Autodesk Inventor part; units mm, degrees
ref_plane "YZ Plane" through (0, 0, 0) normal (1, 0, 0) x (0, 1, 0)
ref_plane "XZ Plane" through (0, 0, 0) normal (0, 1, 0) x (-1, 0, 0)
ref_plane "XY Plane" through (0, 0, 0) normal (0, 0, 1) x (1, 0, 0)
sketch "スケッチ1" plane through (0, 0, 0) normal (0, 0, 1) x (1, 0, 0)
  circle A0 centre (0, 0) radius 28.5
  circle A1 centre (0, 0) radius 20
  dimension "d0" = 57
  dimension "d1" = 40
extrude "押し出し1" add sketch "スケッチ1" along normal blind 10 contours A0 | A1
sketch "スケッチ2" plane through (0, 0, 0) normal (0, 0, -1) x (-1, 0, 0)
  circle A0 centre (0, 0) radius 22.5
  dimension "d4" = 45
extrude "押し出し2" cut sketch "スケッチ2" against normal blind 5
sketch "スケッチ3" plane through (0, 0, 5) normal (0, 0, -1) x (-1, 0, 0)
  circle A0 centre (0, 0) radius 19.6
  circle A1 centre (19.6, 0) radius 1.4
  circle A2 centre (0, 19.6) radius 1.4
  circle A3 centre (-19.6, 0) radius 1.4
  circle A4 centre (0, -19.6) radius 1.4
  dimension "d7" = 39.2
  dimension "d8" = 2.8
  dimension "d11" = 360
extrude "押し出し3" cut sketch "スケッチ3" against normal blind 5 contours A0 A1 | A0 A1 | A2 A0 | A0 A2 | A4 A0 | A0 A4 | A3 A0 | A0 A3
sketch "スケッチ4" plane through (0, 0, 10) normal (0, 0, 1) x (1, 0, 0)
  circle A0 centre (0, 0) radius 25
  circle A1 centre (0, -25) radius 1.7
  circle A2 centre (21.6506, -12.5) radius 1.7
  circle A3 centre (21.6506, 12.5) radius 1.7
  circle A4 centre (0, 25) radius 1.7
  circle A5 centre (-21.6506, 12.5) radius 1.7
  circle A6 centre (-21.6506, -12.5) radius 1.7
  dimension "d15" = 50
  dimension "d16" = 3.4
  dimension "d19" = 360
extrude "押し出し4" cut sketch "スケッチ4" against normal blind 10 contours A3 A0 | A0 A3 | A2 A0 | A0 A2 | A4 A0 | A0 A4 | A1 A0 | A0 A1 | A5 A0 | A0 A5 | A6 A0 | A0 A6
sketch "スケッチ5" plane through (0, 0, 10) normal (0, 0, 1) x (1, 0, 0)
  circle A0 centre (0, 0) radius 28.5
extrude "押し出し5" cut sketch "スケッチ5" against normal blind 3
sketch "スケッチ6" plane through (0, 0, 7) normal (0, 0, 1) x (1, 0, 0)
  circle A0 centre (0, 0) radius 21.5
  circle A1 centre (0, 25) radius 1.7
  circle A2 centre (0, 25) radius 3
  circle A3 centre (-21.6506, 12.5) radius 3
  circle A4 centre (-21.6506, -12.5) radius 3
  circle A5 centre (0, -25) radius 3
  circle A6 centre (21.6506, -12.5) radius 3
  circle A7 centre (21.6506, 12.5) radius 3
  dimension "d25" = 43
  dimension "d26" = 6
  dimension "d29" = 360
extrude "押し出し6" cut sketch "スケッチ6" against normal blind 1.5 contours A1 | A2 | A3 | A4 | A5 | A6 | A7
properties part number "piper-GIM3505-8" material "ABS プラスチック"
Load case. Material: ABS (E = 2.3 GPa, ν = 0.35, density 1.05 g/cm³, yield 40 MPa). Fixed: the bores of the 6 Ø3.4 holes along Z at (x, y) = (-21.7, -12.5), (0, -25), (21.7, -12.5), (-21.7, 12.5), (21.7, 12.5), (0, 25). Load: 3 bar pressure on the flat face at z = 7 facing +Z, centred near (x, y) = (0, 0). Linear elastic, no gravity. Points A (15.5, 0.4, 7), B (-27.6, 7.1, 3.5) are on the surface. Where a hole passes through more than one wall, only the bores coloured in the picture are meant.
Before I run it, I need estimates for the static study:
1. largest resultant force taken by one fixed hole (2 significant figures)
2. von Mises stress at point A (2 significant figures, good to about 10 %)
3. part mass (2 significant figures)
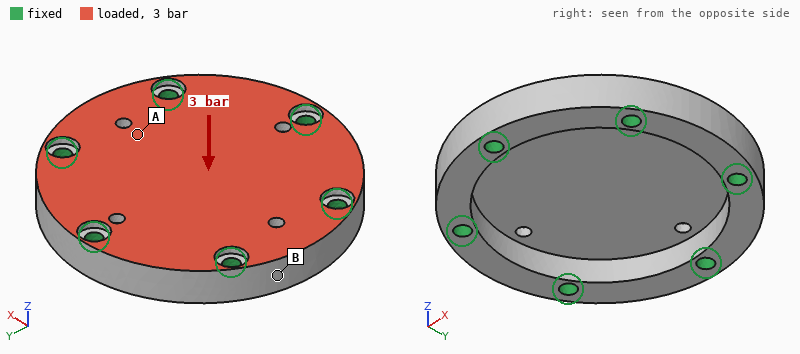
150 N
11 MPa
9.8 g
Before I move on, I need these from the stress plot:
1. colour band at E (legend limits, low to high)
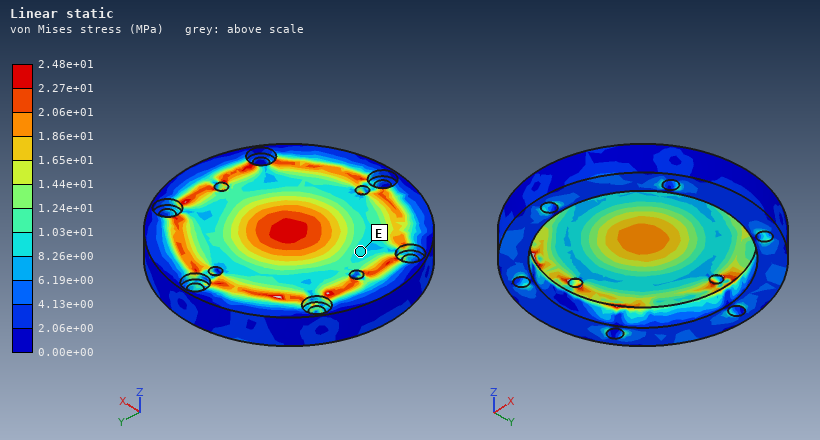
8.26e+00 to 1.03e+01 MPa
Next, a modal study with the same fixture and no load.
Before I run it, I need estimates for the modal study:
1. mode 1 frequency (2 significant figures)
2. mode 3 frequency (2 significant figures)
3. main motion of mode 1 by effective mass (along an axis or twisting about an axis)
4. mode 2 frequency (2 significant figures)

2500 Hz
4900 Hz
along Z
4900 Hz
